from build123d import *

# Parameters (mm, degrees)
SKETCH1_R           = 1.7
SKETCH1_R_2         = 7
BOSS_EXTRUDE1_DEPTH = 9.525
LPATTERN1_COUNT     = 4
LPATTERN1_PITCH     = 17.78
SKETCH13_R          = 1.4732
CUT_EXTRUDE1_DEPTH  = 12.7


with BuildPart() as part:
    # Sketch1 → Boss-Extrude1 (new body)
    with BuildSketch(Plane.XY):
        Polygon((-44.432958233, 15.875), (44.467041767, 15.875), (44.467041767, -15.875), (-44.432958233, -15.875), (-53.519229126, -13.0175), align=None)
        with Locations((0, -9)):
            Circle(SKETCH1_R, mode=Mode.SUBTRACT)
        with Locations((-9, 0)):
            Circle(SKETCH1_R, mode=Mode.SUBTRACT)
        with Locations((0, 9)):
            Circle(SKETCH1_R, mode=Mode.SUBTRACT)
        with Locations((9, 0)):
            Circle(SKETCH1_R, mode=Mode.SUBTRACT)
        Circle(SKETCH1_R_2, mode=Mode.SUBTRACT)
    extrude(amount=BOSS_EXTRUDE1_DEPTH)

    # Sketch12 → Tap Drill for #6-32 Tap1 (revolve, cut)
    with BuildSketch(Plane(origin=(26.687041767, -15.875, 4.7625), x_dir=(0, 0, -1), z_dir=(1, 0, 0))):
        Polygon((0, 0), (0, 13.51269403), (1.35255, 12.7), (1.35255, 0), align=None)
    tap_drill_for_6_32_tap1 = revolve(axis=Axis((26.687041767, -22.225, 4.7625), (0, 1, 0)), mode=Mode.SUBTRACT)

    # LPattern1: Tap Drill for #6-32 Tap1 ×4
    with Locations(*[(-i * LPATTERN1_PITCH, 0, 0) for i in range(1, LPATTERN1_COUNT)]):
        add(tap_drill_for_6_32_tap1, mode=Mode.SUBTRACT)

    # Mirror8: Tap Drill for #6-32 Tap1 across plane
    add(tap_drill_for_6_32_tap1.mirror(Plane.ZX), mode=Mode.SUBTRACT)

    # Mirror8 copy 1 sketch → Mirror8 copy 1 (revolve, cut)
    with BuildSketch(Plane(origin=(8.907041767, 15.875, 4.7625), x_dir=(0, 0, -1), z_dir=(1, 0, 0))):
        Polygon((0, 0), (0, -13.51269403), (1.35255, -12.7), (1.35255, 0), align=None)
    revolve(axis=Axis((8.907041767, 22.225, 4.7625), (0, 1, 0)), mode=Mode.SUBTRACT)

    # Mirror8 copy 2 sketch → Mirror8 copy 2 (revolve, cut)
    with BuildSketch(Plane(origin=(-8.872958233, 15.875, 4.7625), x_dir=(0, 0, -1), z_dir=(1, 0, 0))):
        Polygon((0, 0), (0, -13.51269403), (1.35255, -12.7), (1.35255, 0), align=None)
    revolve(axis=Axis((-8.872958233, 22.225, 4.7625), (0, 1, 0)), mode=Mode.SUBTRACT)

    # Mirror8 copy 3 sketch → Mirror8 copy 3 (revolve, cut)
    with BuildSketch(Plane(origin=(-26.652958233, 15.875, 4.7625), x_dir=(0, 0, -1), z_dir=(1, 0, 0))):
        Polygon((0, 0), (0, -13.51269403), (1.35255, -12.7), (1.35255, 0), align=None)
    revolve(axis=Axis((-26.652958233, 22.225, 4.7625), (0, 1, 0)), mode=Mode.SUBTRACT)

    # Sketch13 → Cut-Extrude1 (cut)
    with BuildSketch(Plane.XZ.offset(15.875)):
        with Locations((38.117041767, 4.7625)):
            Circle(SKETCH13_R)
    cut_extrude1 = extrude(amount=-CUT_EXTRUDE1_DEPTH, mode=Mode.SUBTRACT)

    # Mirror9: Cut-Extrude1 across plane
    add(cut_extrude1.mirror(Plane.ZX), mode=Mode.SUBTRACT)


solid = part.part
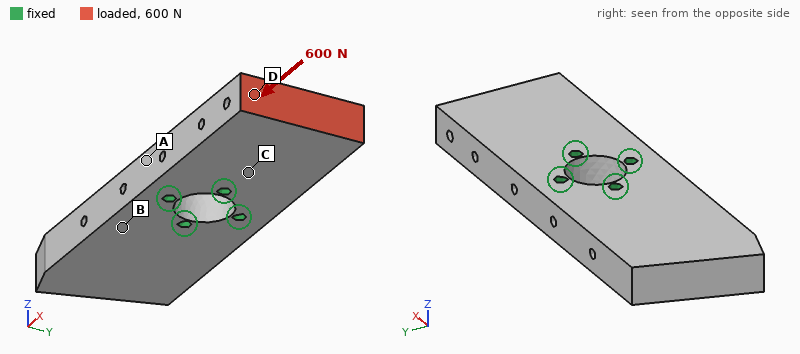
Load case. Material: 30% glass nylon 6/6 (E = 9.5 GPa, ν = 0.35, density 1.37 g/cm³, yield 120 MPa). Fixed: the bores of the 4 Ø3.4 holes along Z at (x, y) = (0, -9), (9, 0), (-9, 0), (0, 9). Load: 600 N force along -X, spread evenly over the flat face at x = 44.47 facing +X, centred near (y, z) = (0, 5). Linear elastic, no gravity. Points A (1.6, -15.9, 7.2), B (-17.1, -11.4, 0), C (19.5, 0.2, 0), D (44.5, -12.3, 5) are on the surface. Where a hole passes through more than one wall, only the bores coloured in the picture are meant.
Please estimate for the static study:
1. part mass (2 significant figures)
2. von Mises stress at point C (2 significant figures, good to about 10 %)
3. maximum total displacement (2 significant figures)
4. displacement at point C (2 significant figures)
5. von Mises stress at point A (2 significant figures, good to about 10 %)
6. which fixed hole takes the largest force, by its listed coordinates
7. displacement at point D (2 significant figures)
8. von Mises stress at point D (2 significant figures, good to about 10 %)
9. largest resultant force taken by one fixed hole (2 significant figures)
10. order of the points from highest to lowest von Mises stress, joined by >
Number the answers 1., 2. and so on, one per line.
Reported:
1. 35 g
2. 2.7 MPa
3. 9.8 µm
4. 3.2 µm
5. 0.92 MPa
6. (9, 0)
7. 9.6 µm
8. 1.6 MPa
9. 300 N
10. C > D > A > B
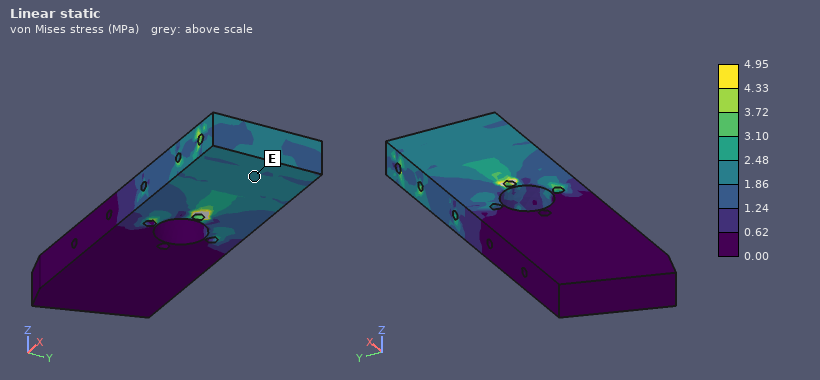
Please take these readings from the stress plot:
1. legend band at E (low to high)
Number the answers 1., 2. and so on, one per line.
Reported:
1. 1.86 to 2.48 MPa
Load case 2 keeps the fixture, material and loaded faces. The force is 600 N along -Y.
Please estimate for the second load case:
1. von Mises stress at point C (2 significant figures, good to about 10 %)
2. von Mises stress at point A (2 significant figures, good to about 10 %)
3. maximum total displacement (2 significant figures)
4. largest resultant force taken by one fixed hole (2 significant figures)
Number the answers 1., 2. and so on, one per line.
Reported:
1. 4.5 MPa
2. 6.9 MPa
3. 0.12 mm
4. 850 N
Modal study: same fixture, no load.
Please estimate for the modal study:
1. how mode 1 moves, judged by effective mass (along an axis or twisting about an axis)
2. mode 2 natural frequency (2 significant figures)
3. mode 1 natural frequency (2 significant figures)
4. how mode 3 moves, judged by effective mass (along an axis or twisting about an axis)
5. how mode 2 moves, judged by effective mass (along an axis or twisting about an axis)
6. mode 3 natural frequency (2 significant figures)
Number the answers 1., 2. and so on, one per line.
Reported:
1. along Z
2. 2700 Hz
3. 2100 Hz
4. along Y
5. along Z
6. 4400 Hz
